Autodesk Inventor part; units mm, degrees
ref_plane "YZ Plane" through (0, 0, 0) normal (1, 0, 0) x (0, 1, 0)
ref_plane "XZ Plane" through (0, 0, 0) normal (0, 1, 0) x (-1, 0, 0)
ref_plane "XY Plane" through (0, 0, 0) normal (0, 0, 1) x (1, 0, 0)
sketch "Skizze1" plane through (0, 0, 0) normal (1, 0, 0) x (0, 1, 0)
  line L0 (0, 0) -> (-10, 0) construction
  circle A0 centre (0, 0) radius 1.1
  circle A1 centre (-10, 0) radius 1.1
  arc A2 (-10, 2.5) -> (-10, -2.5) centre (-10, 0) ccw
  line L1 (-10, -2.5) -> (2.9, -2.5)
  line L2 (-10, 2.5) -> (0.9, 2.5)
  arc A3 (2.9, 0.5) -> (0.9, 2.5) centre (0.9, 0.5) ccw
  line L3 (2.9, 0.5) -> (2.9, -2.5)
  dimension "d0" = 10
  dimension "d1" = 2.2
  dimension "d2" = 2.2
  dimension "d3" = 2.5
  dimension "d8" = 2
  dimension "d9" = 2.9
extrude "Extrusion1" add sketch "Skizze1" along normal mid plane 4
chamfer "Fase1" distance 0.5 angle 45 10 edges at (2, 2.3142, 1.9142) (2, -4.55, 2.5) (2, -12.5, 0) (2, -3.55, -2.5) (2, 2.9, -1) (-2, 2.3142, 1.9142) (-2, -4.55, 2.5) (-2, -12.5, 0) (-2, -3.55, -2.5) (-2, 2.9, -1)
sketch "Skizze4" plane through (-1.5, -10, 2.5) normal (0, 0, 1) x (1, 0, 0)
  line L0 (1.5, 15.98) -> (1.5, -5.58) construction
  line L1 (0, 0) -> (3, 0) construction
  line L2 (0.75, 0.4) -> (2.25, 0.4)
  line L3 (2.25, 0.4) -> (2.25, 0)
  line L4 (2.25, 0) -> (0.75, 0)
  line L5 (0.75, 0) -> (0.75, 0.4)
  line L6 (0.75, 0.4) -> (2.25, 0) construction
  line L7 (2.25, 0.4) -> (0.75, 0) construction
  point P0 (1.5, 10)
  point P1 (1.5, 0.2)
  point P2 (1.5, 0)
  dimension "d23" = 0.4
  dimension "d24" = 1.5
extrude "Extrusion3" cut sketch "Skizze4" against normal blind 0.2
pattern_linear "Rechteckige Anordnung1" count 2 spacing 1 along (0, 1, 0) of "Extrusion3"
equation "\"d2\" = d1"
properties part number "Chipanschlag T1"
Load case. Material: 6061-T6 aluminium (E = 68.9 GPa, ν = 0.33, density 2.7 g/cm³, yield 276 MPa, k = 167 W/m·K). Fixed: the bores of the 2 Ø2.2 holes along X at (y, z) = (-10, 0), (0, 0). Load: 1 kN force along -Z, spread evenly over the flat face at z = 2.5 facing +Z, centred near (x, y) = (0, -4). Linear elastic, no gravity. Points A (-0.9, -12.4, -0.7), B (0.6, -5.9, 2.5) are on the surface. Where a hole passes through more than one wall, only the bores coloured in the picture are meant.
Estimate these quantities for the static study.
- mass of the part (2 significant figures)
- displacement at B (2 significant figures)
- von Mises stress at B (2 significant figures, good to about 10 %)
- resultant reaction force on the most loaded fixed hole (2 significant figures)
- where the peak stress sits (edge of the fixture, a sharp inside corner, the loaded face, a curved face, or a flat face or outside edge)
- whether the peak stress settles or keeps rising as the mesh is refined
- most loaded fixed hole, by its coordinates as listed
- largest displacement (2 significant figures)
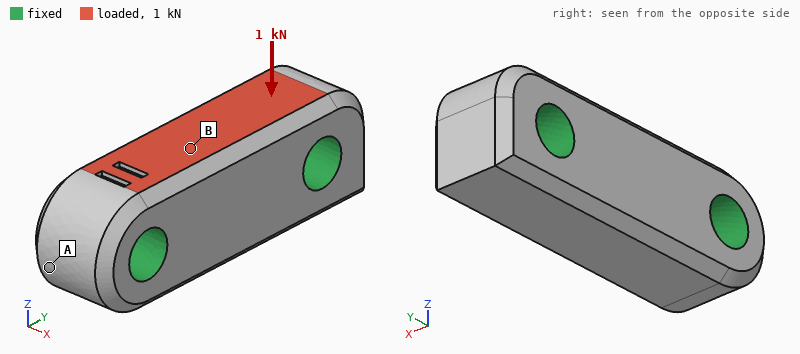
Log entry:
0.69 g
3.4 µm
29 MPa
570 N
edge of the fixture
keeps rising
(0, 0)
3.6 µm
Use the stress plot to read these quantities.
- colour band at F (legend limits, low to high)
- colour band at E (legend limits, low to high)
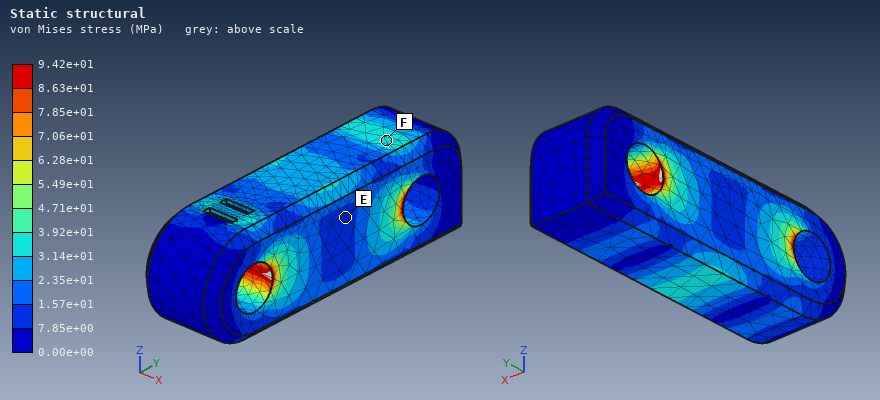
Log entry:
3.14e+01 to 3.92e+01 MPa
7.85e+00 to 1.57e+01 MPa
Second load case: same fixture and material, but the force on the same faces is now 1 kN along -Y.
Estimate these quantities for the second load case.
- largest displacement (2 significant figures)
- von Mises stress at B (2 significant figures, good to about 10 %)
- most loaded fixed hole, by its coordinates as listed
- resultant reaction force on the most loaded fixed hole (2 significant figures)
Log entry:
2.5 µm
56 MPa
(0, 0)
580 N
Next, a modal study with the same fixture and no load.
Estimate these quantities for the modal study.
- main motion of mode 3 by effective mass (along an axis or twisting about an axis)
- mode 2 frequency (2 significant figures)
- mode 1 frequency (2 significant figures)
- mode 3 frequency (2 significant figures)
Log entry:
twisting about Y
140 kHz
140 kHz
160 kHz
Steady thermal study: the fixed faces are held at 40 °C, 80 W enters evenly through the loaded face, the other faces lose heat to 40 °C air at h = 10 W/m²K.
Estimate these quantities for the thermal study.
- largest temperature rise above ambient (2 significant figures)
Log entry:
46 K
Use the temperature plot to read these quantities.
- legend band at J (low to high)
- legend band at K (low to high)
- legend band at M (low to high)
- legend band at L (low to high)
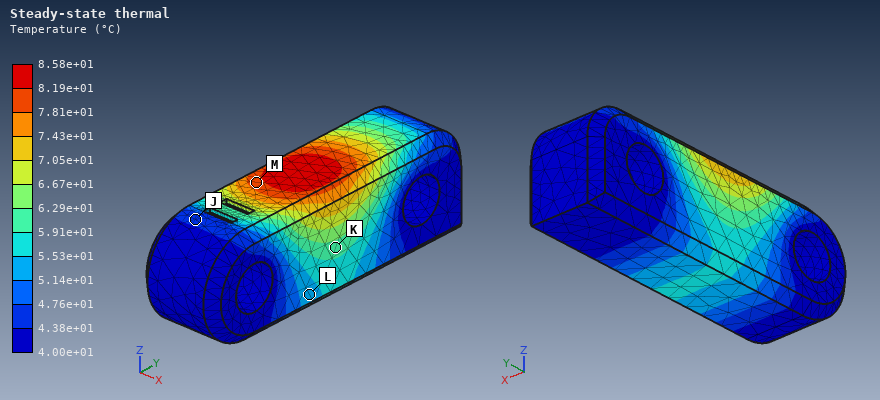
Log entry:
4.38e+01 to 4.76e+01 °C
5.91e+01 to 6.29e+01 °C
7.81e+01 to 8.19e+01 °C
5.14e+01 to 5.53e+01 °C
